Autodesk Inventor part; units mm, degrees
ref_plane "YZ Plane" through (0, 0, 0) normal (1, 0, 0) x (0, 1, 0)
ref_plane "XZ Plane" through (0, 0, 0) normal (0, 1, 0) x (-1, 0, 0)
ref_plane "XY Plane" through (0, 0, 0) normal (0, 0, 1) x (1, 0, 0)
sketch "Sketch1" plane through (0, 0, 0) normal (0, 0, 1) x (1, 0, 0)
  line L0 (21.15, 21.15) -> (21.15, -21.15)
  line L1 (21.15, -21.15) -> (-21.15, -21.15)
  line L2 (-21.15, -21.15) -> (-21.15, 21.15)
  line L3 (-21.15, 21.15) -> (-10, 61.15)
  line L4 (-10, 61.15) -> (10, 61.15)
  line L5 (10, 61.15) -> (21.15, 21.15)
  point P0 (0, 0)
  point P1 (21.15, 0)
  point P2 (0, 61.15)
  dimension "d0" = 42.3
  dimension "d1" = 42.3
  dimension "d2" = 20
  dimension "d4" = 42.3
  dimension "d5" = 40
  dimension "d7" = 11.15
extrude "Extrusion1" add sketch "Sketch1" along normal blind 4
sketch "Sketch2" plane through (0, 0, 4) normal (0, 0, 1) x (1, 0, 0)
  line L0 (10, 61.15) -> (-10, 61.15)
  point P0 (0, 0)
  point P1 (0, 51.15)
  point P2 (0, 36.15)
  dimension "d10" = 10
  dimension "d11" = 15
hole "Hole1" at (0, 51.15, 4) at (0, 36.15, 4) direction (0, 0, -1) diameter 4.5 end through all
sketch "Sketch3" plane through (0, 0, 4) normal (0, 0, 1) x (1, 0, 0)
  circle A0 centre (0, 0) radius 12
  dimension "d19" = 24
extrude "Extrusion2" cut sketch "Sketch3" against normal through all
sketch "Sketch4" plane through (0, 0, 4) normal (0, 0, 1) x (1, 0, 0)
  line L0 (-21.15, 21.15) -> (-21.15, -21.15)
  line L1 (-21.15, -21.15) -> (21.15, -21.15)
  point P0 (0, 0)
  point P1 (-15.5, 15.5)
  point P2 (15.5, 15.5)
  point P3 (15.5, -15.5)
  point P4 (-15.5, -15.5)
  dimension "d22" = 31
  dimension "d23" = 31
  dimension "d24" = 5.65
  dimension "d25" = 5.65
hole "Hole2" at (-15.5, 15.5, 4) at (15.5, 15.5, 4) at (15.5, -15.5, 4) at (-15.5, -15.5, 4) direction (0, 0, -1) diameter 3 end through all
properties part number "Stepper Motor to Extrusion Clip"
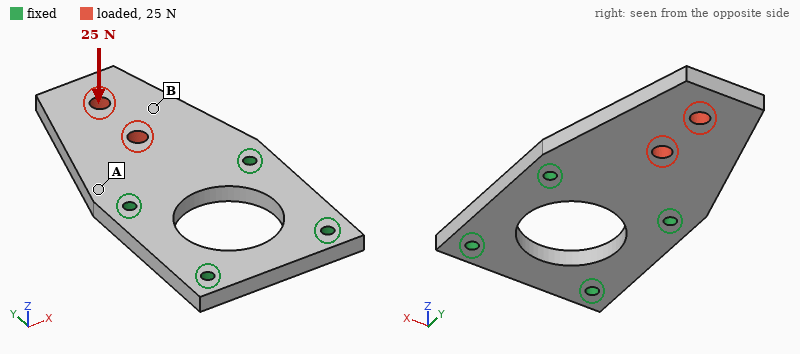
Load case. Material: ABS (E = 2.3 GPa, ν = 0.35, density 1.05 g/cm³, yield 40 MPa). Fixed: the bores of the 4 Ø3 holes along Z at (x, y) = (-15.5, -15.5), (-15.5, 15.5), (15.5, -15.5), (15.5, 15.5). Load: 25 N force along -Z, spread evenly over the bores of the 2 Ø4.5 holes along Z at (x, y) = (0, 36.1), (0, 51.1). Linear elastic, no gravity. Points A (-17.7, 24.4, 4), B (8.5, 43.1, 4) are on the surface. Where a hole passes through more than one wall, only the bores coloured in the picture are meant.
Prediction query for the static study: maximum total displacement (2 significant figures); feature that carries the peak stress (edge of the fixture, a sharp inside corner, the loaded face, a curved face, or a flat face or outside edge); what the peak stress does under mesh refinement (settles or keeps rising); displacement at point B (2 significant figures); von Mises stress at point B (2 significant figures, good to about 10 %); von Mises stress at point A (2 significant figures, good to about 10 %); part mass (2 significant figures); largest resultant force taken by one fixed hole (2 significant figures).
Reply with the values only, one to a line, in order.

0.97 mm
edge of the fixture
keeps rising
0.47 mm
1.8 MPa
5.3 MPa
11 g
15 N
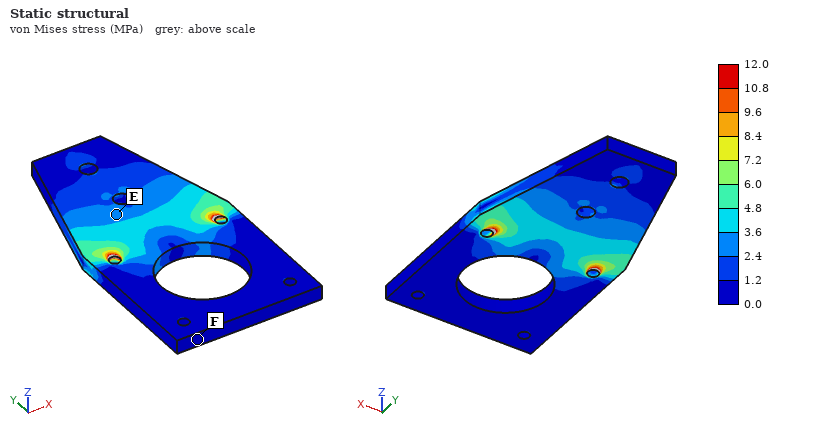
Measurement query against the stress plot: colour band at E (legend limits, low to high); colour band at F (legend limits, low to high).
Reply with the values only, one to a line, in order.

2.4 to 3.6 MPa
0.0 to 1.2 MPa
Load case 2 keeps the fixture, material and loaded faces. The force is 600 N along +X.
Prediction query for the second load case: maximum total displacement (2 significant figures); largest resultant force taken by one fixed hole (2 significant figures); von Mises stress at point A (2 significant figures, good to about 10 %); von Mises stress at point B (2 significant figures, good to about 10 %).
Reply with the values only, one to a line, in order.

0.37 mm
570 N
9.8 MPa
4.3 MPa
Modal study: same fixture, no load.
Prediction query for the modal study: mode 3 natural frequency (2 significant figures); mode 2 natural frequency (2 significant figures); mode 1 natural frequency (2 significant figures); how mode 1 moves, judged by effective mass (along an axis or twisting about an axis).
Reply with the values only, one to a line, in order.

2700 Hz
2000 Hz
530 Hz
along Z
